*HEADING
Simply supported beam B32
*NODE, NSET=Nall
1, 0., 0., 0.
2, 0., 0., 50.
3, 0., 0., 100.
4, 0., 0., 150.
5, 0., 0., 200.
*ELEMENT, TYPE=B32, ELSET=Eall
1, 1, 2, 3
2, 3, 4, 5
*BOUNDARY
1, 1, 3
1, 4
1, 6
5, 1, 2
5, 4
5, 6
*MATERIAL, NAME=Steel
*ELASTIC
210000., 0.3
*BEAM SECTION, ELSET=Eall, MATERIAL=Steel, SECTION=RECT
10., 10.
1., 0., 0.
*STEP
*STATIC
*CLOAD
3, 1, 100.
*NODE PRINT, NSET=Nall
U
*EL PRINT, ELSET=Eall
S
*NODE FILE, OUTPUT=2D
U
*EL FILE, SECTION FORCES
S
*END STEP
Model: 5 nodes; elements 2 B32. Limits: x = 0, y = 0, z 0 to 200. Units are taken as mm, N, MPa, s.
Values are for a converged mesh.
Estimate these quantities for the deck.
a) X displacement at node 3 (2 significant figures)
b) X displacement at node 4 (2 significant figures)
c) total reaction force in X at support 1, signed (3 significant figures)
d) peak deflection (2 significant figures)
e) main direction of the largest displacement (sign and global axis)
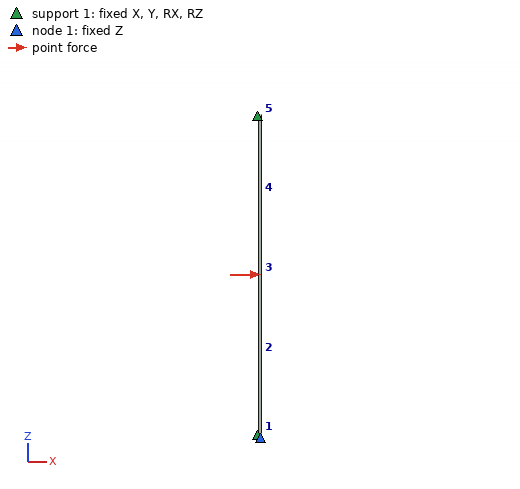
0.096 mm
0.066 mm
-100 N
0.096 mm
+X
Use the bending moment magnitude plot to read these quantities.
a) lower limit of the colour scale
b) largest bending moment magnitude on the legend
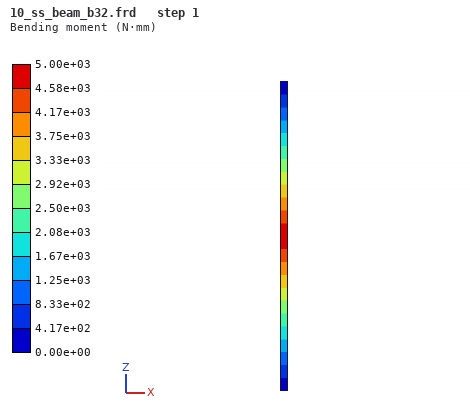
0.00e+00 N·mm
5.00e+03 N·mm
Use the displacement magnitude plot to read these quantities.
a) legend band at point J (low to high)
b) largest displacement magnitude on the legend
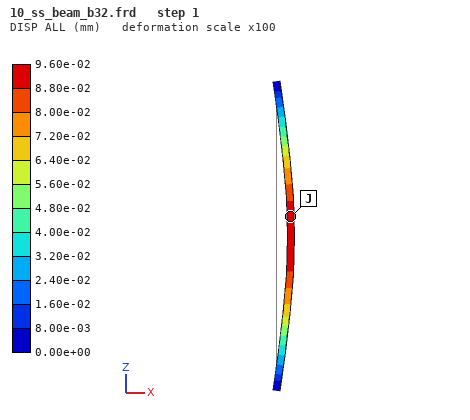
8.80e-02 to 9.60e-02 mm
9.60e-02 mm
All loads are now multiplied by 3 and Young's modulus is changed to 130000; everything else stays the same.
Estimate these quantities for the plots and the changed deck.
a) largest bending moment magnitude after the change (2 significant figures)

15000 N·mm
